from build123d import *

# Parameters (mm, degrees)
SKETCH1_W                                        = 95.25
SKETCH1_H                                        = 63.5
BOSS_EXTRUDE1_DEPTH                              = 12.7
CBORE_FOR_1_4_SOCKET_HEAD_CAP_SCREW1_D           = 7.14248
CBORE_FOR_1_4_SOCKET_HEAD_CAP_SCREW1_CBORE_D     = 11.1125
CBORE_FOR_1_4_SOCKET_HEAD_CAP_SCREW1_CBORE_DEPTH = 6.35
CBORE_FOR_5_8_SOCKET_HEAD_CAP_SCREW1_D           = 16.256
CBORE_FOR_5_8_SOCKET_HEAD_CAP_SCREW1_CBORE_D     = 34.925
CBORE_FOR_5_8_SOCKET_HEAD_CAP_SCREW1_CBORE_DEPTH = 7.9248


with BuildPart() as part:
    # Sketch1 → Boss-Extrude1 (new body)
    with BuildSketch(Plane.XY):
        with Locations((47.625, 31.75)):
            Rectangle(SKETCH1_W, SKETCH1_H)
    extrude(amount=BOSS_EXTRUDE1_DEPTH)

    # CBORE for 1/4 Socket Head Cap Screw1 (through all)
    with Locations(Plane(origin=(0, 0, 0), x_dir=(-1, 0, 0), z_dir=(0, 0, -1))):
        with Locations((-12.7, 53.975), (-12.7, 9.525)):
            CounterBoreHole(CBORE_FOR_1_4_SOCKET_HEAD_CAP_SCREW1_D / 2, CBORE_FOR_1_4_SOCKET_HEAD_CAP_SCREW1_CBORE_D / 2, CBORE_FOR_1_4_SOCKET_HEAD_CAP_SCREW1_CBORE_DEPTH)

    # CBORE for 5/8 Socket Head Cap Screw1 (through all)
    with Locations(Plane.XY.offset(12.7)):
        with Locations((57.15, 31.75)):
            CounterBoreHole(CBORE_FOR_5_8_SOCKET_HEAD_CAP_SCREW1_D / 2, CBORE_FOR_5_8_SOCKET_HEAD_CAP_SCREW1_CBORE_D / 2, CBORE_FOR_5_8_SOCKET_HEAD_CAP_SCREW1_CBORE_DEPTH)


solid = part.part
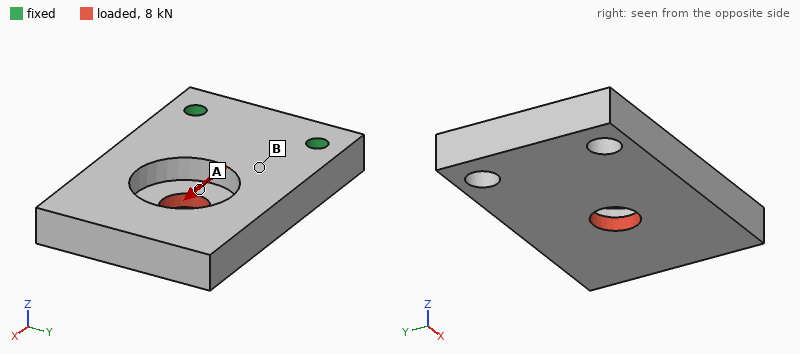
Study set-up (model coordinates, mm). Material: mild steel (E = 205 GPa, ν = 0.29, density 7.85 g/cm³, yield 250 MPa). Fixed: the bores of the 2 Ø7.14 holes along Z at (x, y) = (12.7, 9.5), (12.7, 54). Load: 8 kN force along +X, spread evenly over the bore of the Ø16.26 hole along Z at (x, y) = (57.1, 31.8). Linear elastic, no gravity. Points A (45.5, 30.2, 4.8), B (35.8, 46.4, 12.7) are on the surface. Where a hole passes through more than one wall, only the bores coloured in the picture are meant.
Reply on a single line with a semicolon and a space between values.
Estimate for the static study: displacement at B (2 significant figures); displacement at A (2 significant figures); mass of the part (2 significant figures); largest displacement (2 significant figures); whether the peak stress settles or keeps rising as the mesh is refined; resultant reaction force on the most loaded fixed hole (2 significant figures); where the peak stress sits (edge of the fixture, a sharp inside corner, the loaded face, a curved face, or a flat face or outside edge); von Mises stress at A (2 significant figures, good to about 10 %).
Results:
17 µm; 27 µm; 520 g; 86 µm; keeps rising; 4.0 kN; edge of the fixture; 32 MPa
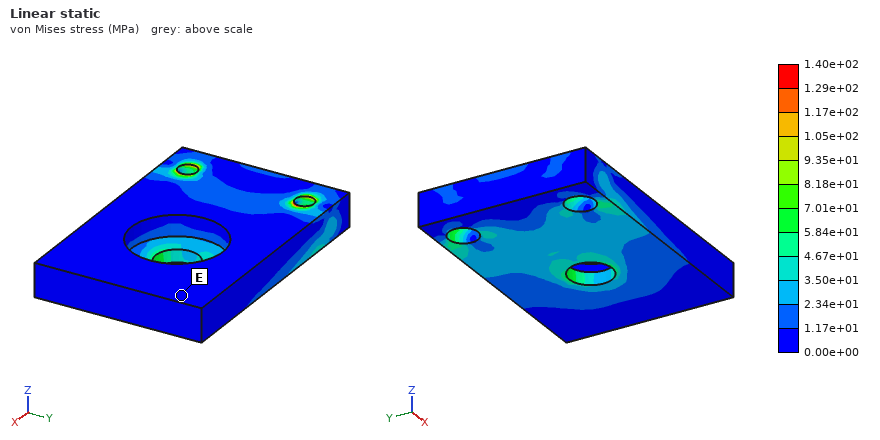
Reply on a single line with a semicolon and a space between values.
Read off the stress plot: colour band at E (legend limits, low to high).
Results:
0.00e+00 to 1.17e+01 MPa
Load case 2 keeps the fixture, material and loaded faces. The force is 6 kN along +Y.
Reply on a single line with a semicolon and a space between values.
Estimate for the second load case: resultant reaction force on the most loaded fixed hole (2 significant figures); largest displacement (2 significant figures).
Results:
6.4 kN; 21 µm
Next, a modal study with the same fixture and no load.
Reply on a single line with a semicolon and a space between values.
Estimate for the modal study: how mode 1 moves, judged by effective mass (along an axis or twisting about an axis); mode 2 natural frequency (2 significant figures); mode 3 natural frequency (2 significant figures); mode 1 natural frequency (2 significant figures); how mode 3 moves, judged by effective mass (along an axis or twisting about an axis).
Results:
along Z; 3400 Hz; 4800 Hz; 1100 Hz; along Y
